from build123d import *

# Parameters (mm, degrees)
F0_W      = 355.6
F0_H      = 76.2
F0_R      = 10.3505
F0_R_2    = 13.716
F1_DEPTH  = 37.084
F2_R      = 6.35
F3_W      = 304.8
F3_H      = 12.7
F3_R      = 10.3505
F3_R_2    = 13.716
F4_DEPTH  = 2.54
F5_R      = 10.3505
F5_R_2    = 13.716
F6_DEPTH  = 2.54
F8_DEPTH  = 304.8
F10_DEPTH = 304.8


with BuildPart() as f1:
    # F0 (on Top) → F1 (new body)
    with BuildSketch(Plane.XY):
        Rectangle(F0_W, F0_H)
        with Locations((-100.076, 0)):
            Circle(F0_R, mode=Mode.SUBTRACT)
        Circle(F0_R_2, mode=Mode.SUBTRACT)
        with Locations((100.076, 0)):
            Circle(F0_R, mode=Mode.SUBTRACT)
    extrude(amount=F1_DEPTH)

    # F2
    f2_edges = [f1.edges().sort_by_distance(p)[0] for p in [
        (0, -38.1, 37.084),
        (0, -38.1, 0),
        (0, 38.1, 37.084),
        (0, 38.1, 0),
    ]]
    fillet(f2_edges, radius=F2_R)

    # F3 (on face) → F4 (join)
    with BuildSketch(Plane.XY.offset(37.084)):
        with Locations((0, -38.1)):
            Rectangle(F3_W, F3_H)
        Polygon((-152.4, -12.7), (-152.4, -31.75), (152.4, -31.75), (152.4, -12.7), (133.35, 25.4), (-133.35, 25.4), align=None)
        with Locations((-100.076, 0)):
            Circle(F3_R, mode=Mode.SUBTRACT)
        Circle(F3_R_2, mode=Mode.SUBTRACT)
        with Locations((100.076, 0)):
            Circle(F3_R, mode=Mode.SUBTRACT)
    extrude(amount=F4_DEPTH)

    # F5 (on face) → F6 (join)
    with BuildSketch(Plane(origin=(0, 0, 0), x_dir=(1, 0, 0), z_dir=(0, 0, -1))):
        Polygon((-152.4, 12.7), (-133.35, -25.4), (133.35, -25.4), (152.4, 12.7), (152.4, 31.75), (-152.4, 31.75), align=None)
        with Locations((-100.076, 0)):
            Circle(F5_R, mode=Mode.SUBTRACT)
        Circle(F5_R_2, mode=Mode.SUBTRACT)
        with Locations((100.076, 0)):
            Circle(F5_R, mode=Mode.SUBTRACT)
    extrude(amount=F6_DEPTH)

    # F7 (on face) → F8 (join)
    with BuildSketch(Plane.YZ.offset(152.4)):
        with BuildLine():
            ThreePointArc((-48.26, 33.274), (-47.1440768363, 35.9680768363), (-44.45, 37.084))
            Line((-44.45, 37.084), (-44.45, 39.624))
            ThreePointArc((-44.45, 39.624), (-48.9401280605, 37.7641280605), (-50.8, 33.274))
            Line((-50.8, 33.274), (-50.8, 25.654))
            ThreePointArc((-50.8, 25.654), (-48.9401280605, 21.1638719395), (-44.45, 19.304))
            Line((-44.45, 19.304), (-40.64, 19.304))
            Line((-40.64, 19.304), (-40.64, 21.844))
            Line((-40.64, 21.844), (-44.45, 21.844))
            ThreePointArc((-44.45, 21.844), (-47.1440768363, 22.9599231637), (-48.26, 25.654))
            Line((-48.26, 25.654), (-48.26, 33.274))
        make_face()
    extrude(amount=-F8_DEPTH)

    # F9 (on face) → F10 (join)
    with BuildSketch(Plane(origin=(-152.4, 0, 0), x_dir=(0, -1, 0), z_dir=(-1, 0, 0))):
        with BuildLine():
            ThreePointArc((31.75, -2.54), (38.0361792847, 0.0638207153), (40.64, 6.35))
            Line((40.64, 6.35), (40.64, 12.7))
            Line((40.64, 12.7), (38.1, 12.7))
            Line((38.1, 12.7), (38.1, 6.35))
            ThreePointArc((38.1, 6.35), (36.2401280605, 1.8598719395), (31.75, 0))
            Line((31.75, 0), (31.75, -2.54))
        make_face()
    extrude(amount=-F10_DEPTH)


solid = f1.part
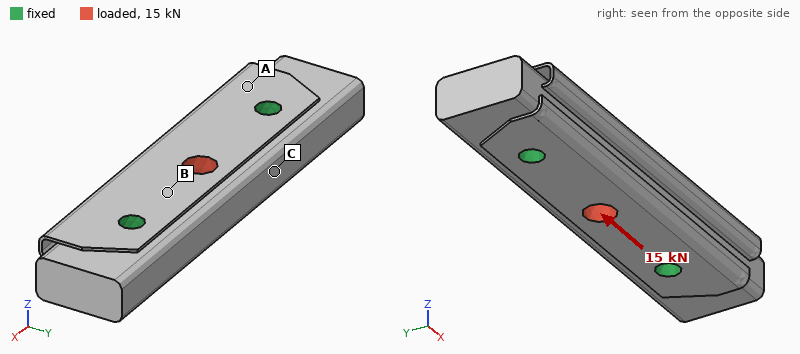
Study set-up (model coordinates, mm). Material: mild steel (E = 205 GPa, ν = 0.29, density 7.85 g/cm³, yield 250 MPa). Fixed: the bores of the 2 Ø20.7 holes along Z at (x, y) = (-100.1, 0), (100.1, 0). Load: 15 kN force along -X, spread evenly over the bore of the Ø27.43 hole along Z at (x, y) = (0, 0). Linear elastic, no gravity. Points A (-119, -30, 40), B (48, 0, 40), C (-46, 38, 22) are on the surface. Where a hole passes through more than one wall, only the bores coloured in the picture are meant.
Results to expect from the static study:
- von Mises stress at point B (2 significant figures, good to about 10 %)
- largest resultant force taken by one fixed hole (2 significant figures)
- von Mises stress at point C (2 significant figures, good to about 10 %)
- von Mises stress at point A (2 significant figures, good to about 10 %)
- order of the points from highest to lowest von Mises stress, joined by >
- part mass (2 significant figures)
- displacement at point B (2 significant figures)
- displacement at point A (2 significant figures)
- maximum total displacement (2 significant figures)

3.3 MPa
7.5 kN
1.9 MPa
0.81 MPa
B > C > A
8.4 kg
0.72 µm
0.23 µm
1.4 µm
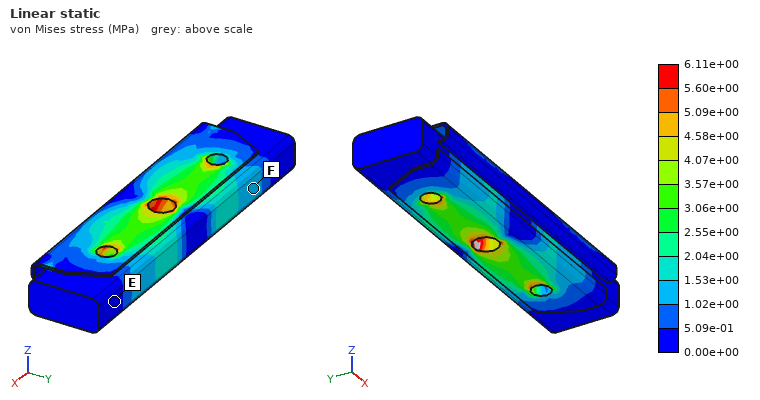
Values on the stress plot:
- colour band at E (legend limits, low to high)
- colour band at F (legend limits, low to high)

0.00e+00 to 5.09e-01 MPa
1.02e+00 to 1.53e+00 MPa
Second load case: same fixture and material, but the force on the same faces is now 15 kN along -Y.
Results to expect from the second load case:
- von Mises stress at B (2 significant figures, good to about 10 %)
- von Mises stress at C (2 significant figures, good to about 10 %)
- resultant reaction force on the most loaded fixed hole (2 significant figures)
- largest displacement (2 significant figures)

5.8 MPa
3.9 MPa
7.5 kN
10 µm
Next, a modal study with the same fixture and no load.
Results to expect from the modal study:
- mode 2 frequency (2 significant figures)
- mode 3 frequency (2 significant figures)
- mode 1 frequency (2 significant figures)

1900 Hz
2800 Hz
1800 Hz
